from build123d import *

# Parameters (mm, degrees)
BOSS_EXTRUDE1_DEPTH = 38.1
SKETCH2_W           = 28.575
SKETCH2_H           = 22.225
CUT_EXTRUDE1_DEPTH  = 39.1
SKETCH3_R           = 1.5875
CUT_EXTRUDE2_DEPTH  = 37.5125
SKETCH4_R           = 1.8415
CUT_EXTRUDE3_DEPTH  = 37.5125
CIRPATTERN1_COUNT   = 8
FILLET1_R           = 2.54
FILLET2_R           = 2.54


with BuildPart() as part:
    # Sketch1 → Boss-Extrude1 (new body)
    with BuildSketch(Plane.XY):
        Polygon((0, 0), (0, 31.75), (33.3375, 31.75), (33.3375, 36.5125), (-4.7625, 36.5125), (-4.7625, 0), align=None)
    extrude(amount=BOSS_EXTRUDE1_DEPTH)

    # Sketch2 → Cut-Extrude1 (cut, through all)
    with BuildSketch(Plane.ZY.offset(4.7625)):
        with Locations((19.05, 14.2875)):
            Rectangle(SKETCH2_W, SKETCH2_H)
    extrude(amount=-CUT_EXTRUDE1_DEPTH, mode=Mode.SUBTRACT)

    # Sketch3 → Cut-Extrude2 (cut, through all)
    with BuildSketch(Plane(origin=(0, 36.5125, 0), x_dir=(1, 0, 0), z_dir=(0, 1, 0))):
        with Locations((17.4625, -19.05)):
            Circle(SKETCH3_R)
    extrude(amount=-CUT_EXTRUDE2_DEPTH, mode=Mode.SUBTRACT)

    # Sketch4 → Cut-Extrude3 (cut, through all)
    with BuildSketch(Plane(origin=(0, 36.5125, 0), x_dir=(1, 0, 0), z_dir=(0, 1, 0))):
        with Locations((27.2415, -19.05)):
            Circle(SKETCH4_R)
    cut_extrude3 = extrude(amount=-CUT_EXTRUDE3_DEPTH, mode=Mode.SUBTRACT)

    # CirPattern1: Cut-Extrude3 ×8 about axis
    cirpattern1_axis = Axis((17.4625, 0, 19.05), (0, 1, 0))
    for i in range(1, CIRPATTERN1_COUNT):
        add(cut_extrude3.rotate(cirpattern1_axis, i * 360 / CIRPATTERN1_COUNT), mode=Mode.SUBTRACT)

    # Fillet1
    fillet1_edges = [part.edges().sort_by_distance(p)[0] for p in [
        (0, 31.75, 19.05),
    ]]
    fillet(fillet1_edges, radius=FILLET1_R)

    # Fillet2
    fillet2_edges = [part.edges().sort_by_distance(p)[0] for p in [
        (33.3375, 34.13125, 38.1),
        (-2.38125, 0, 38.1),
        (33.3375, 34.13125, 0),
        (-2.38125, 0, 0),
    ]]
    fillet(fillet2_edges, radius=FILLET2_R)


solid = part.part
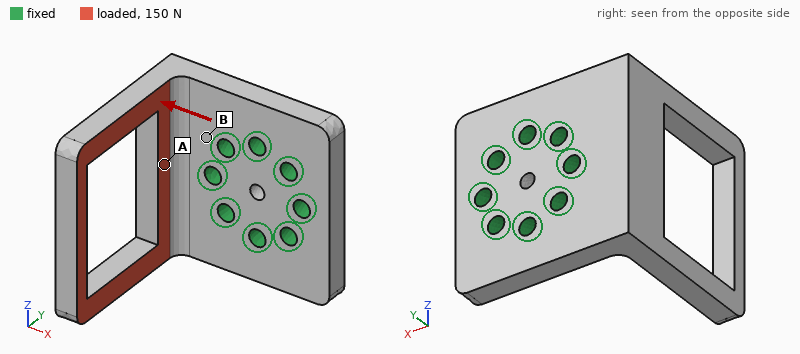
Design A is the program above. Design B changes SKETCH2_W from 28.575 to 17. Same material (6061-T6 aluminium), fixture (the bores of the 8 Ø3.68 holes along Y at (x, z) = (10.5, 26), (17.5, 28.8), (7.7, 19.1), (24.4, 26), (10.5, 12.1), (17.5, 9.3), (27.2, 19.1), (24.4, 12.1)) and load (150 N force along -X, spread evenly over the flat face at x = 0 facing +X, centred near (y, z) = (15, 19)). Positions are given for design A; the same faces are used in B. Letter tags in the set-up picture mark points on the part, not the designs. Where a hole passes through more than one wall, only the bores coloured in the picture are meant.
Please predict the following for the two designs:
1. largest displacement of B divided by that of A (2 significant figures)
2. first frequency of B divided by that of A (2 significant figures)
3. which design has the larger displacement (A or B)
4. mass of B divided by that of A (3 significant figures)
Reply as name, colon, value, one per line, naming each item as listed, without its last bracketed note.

largest displacement of B divided by that of A: 0.61
first frequency of B divided by that of A: 1.1
which design has the larger displacement: A
mass of B divided by that of A: 1.13
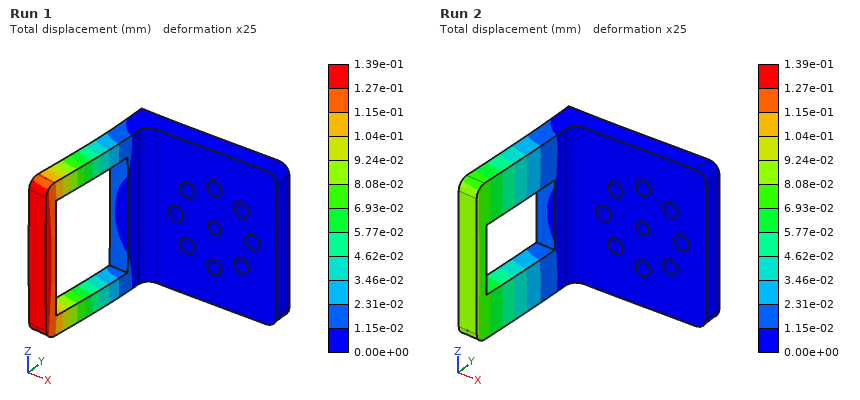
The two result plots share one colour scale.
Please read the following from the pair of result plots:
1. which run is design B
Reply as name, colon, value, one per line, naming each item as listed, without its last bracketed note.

which run is design B: Run 2
